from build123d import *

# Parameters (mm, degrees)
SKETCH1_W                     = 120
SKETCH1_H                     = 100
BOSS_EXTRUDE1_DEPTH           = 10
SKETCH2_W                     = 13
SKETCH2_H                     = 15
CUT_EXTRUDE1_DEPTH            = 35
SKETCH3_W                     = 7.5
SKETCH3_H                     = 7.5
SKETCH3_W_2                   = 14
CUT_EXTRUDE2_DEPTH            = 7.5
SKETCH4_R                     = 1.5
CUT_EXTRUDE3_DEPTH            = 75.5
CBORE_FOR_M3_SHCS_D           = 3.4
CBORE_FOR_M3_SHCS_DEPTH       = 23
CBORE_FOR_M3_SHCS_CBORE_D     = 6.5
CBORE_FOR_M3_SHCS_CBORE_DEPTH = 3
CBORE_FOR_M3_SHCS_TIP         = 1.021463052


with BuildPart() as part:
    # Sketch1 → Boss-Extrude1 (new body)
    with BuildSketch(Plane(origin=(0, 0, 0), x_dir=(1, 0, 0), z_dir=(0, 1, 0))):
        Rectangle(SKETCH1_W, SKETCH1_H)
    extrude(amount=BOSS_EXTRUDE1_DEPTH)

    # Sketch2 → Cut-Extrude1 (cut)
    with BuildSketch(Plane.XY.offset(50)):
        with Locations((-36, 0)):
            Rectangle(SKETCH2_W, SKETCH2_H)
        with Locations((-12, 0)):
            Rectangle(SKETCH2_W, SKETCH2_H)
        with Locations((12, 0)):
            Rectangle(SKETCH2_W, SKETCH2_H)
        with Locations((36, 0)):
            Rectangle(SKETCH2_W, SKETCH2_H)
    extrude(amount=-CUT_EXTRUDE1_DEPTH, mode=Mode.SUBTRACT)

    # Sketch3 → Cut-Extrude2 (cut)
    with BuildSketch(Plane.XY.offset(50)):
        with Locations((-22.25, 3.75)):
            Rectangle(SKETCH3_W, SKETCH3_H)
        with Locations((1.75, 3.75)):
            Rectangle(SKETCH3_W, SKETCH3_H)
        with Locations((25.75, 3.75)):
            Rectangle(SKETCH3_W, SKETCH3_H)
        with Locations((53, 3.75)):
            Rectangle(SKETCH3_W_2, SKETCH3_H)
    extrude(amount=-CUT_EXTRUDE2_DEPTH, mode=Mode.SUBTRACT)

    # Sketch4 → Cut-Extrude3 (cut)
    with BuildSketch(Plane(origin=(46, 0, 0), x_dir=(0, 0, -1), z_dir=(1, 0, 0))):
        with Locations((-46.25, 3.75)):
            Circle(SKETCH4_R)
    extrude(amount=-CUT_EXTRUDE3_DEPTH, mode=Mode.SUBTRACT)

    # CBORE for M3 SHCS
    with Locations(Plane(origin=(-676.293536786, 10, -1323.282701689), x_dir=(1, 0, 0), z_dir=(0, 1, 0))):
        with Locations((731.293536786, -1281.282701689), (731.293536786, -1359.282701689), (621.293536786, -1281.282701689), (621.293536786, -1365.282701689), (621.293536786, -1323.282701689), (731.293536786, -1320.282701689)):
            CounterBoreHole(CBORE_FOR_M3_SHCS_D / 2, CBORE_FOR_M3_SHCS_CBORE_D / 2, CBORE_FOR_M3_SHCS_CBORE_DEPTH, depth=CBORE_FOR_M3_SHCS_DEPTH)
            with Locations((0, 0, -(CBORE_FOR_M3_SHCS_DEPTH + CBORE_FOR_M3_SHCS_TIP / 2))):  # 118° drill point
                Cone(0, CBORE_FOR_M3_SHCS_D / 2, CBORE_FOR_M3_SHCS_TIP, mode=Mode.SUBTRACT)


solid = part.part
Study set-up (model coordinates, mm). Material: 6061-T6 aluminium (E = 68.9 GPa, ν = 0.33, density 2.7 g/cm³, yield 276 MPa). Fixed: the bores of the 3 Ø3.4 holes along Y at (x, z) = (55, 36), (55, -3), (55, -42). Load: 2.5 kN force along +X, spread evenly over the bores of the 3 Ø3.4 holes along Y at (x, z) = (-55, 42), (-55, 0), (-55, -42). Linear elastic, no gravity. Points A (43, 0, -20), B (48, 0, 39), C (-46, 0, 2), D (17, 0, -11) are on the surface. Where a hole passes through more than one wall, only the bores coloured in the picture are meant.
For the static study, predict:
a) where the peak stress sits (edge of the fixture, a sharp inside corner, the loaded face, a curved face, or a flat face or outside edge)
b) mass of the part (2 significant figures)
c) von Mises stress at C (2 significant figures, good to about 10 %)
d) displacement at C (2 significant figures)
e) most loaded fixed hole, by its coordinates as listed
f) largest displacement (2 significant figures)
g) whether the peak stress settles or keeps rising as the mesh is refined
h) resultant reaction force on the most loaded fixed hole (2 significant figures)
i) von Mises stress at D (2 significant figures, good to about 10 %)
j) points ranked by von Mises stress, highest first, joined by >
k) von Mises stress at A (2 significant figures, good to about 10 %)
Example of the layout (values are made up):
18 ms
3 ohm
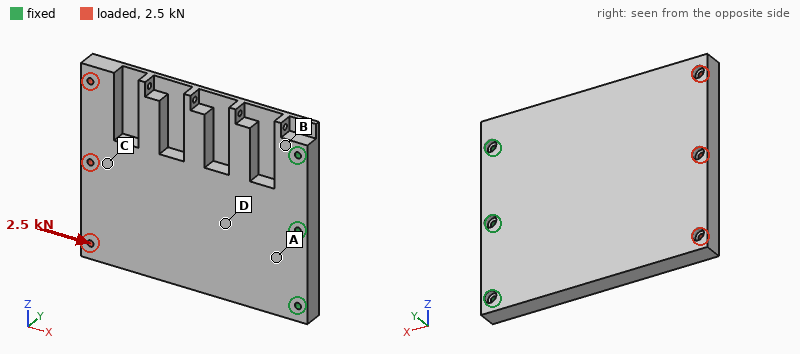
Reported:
edge of the fixture
280 g
11 MPa
0.081 mm
(55, -3)
0.13 mm
keeps rising
1.4 kN
8.4 MPa
C > D > A > B
4.5 MPa
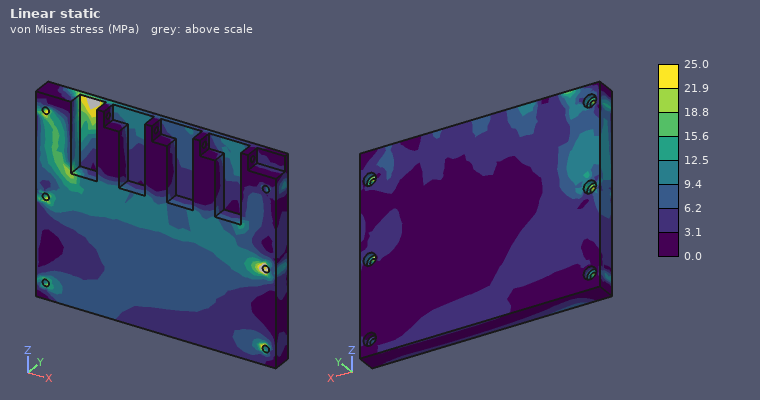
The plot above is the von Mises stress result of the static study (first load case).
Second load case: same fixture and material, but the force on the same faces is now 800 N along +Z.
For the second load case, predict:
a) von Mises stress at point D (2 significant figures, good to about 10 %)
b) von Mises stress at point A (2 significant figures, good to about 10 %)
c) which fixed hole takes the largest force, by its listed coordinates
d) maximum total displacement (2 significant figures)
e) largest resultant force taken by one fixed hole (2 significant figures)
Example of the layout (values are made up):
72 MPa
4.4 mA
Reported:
3.9 MPa
3.8 MPa
(55, -42)
54 µm
1.4 kN
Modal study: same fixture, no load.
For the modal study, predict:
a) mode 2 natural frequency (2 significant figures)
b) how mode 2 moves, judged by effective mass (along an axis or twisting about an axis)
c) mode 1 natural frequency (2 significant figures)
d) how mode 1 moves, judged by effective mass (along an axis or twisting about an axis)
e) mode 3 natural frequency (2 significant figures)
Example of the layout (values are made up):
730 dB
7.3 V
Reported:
1400 Hz
twisting about X
440 Hz
along Y
2700 Hz
